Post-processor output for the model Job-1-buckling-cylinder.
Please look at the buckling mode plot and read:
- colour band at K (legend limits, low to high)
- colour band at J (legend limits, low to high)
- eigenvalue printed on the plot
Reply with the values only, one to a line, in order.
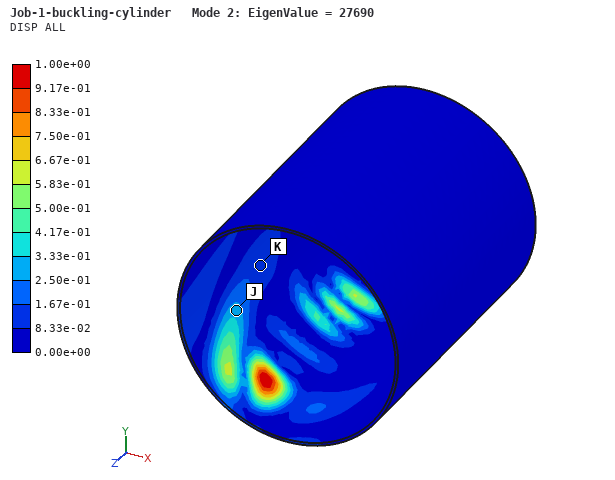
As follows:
8.33e-02 to 1.67e-01
2.50e-01 to 3.33e-01
27690
